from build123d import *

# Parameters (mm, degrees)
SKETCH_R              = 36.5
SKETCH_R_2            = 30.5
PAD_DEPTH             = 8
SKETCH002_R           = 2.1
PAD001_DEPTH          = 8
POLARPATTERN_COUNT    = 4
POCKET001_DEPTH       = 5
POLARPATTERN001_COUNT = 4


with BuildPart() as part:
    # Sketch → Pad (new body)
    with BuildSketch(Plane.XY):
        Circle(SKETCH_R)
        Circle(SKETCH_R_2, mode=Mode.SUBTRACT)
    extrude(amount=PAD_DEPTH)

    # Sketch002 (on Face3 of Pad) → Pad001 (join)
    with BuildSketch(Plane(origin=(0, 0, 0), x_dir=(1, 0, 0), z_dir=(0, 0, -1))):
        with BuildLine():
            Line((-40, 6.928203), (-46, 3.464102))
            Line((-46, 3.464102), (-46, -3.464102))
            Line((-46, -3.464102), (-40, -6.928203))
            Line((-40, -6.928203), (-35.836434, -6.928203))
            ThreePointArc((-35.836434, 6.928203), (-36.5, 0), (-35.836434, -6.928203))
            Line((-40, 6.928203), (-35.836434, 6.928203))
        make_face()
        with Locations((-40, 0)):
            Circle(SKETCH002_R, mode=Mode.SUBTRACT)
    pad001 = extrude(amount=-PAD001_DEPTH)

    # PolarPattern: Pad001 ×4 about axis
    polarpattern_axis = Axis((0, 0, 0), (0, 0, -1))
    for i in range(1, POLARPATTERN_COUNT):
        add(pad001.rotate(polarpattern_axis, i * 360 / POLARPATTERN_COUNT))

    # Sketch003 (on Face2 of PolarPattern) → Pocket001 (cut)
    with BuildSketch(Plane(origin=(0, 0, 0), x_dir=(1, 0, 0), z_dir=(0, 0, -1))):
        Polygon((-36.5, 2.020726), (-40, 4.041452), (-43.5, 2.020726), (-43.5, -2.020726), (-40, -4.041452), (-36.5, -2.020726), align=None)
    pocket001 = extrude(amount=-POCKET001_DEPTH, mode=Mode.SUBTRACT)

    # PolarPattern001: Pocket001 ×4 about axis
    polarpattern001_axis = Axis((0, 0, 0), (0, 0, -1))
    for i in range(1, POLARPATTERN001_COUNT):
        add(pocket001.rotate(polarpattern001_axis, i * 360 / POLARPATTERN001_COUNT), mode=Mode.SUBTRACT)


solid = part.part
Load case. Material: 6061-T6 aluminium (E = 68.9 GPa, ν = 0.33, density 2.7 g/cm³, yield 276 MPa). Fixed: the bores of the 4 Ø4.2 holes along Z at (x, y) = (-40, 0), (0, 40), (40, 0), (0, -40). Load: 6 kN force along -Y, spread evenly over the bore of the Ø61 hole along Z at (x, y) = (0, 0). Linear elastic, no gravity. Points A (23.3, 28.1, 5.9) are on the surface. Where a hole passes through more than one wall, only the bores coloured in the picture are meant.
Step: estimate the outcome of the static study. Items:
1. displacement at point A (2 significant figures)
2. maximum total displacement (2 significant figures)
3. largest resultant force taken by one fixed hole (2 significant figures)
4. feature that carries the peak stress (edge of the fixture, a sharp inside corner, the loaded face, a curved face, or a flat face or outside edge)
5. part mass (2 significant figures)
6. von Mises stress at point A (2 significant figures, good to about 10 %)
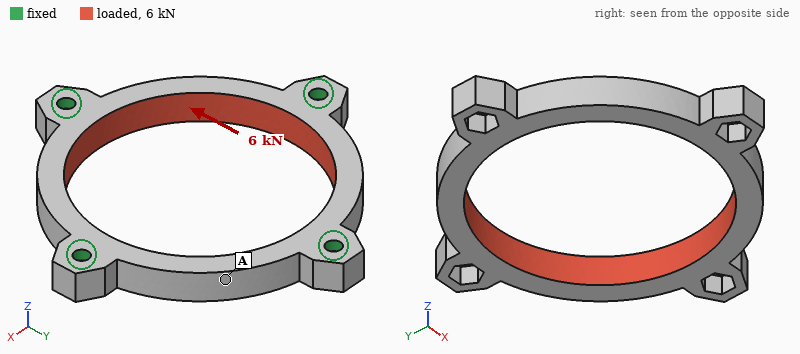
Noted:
28 µm
35 µm
2.1 kN
edge of the fixture
34 g
27 MPa
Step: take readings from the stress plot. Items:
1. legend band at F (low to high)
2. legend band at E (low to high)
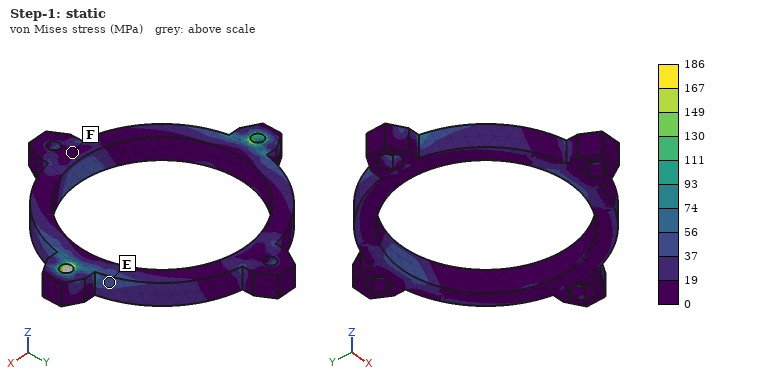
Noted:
0 to 19 MPa
37 to 56 MPa
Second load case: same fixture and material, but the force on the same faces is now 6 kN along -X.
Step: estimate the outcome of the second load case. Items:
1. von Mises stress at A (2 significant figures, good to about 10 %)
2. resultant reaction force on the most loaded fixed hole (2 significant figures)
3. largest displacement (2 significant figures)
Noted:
33 MPa
2.1 kN
35 µm
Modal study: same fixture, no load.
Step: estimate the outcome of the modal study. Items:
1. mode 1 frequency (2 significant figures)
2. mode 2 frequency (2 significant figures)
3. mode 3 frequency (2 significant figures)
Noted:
7500 Hz
9100 Hz
9100 Hz
